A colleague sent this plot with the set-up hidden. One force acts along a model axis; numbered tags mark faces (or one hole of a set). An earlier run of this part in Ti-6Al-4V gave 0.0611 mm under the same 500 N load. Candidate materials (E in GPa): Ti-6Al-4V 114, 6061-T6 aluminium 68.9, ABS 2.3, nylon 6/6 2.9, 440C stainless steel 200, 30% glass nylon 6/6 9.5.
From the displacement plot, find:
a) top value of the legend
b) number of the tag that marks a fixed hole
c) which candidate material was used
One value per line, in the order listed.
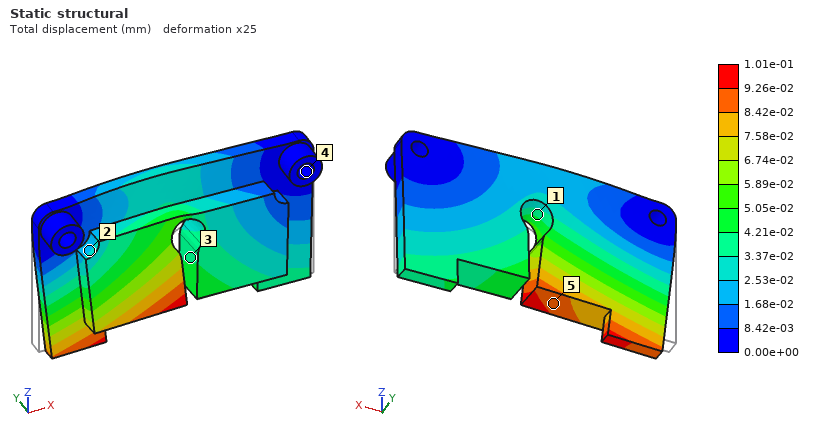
1.01e-01 mm
4
6061-T6 aluminium
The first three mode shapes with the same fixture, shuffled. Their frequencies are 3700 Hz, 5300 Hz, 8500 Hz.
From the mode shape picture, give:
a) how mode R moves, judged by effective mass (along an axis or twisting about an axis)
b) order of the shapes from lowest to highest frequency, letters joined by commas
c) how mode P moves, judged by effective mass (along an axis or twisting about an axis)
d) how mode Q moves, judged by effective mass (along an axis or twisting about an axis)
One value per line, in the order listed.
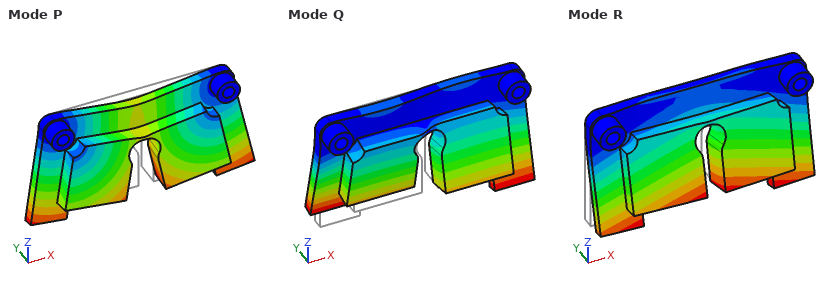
along Y
R, Q, P
along Z
twisting about Z
